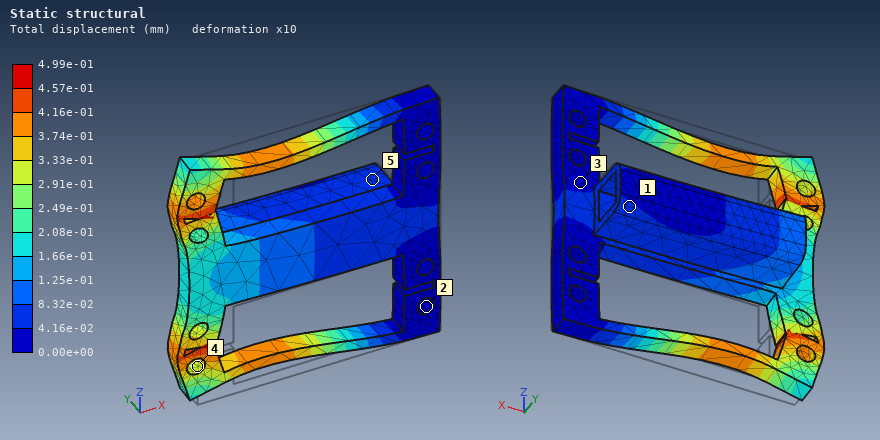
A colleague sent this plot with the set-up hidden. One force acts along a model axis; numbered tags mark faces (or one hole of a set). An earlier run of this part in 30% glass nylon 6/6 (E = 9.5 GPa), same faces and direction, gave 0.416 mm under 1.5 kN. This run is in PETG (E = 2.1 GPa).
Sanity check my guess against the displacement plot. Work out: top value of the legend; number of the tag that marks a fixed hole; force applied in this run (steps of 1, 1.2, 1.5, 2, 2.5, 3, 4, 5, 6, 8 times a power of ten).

4.99e-01 mm
2
400 N
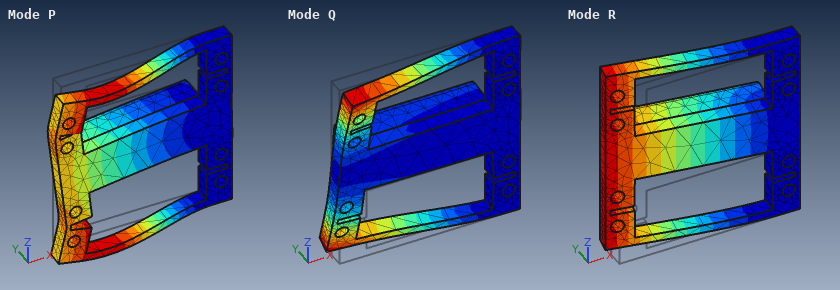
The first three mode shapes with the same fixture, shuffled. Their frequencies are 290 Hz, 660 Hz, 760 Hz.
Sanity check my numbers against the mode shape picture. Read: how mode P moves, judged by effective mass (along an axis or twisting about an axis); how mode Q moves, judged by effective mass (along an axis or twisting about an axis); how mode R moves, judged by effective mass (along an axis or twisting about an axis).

along Z
twisting about X
along Y
